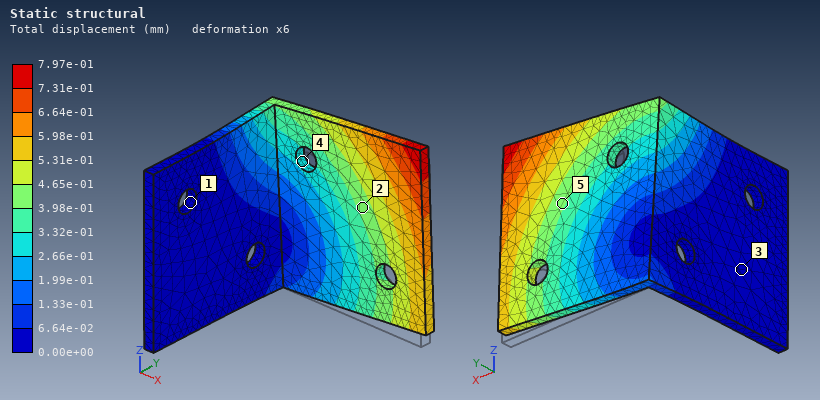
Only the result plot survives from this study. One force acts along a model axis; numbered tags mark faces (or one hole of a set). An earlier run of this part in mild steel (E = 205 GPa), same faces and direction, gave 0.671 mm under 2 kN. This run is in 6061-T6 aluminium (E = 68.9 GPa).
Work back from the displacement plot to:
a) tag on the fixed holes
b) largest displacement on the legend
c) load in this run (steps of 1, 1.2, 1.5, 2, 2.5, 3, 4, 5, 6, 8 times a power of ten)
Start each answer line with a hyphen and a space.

- 1
- 7.97e-01 mm
- 800 N
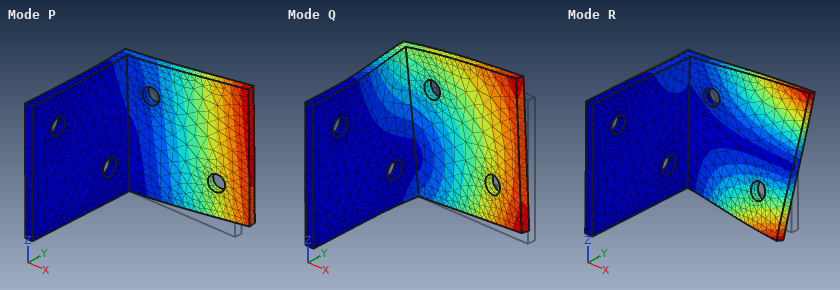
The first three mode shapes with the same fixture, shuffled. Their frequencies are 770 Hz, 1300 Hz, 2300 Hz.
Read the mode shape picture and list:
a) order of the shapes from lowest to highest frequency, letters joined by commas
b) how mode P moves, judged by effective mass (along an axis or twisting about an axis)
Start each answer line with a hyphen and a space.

- P, Q, R
- along Y
